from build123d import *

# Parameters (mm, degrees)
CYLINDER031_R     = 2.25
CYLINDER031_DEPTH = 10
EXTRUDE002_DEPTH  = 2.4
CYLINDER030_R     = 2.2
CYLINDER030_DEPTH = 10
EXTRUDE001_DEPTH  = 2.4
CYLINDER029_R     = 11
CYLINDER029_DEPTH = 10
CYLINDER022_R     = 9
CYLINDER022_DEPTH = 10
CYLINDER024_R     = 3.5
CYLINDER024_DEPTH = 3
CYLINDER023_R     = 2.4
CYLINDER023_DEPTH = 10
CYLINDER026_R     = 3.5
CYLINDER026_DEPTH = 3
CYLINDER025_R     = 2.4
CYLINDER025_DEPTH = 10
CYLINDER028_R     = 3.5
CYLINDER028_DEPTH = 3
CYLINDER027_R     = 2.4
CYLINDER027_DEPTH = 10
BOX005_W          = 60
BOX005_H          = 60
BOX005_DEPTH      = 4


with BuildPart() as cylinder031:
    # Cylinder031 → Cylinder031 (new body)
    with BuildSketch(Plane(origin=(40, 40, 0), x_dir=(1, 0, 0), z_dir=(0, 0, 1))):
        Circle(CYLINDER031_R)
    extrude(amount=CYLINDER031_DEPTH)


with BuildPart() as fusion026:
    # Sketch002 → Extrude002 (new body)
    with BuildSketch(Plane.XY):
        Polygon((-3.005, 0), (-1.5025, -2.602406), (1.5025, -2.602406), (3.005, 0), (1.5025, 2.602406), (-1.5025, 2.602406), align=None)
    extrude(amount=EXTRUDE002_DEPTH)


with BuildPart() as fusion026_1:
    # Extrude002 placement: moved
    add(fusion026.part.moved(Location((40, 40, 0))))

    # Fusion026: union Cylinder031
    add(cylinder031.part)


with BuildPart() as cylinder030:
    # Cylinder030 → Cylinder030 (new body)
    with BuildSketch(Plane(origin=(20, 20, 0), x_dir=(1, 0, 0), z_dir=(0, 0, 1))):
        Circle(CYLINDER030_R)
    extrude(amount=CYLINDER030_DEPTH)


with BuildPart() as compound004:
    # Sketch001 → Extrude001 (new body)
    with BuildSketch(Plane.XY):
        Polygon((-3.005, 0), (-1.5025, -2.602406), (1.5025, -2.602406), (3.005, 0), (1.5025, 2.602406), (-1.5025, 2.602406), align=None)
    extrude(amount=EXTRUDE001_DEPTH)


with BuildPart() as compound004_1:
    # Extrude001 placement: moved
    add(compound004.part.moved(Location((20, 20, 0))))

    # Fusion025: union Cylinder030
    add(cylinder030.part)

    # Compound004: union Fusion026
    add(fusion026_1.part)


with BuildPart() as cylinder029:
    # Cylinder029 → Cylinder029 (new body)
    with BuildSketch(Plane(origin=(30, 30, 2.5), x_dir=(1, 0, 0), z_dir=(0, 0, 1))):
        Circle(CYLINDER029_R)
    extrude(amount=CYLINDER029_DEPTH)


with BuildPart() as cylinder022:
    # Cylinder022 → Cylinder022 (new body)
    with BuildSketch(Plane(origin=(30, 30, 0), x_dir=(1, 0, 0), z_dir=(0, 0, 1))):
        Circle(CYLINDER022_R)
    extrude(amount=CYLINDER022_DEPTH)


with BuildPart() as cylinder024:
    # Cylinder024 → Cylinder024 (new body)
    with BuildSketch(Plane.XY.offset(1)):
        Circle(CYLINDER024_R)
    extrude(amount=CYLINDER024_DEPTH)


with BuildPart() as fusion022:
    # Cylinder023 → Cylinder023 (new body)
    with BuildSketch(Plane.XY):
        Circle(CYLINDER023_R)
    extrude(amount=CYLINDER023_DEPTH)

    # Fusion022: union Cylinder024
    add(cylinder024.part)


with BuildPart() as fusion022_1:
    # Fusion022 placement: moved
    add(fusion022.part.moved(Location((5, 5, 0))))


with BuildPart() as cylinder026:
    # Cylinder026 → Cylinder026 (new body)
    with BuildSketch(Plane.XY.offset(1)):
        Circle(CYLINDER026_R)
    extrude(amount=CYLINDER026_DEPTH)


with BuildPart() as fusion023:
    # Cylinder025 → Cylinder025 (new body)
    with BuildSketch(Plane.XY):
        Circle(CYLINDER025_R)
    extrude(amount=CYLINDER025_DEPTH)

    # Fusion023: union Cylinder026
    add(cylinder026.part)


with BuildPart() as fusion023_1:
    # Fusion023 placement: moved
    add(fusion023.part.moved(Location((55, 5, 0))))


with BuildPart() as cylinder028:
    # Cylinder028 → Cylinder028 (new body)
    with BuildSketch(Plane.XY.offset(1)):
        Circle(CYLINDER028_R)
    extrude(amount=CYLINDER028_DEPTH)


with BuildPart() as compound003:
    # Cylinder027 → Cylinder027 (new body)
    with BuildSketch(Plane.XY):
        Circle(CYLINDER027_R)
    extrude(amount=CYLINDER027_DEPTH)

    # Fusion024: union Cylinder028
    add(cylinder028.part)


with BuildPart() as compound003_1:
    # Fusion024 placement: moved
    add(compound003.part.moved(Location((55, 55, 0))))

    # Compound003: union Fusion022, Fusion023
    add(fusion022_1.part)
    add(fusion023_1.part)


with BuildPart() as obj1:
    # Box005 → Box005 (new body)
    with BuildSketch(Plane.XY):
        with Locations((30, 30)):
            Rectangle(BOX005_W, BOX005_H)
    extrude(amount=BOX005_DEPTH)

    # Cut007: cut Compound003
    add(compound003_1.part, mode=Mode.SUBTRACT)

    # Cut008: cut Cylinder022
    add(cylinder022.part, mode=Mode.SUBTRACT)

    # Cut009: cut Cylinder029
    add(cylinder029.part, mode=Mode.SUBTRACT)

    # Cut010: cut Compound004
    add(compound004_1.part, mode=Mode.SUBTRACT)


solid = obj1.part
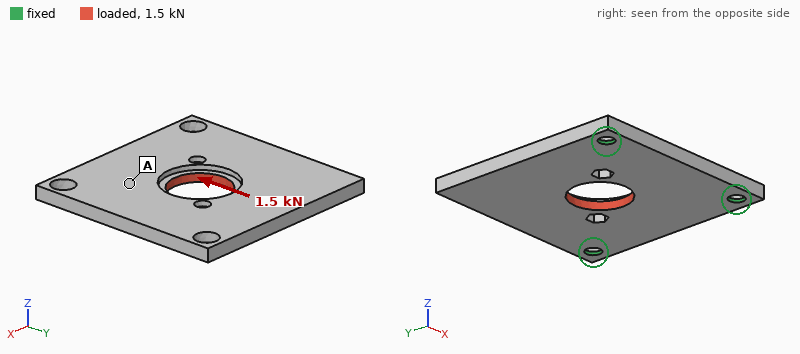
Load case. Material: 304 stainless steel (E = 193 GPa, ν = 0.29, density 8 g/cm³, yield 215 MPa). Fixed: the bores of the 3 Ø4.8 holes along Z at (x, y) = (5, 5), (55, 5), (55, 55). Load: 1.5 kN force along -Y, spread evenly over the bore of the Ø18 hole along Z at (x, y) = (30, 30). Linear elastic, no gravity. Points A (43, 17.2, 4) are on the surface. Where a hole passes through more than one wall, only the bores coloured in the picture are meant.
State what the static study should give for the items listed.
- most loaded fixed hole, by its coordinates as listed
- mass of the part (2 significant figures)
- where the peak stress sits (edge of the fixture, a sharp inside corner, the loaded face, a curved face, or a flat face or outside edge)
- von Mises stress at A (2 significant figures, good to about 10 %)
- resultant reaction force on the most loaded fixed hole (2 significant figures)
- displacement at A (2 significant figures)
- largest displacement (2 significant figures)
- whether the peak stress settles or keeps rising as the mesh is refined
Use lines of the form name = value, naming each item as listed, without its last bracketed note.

most loaded fixed hole, by its coordinates as listed = (5, 5)
mass of the part = 100 g
where the peak stress sits = edge of the fixture
von Mises stress at A = 7.5 MPa
resultant reaction force on the most loaded fixed hole = 620 N
displacement at A = 2.5 µm
largest displacement = 3.9 µm
whether the peak stress settles or keeps rising as the mesh is refined = keeps rising
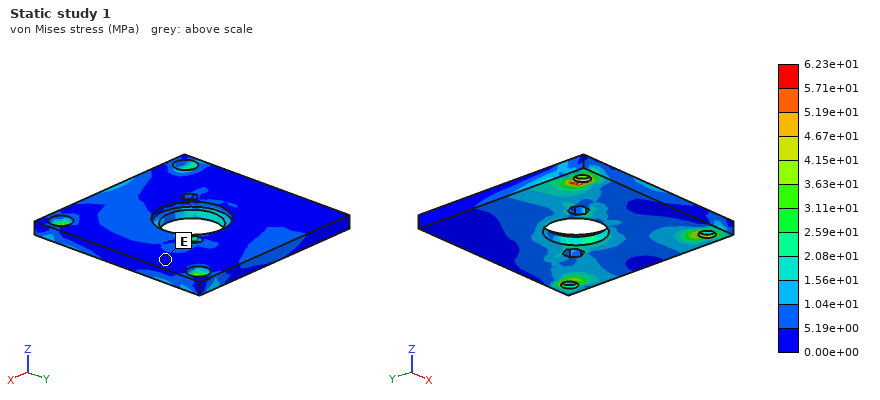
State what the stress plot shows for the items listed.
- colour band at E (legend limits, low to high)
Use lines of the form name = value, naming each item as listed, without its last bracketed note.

colour band at E = 0.00e+00 to 5.19e+00 MPa
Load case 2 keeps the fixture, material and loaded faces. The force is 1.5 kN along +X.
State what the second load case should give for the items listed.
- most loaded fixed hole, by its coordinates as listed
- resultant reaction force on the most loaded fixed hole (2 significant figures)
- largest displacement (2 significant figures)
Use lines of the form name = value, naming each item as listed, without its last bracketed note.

most loaded fixed hole, by its coordinates as listed = (55, 55)
resultant reaction force on the most loaded fixed hole = 620 N
largest displacement = 3.9 µm
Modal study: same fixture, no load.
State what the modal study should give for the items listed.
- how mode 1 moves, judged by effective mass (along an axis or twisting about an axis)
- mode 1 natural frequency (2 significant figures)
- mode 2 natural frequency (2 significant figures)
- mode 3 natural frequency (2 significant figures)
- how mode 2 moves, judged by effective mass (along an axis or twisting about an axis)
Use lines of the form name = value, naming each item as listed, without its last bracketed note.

how mode 1 moves, judged by effective mass = along Z
mode 1 natural frequency = 1500 Hz
mode 2 natural frequency = 4600 Hz
mode 3 natural frequency = 5700 Hz
how mode 2 moves, judged by effective mass = along Z
